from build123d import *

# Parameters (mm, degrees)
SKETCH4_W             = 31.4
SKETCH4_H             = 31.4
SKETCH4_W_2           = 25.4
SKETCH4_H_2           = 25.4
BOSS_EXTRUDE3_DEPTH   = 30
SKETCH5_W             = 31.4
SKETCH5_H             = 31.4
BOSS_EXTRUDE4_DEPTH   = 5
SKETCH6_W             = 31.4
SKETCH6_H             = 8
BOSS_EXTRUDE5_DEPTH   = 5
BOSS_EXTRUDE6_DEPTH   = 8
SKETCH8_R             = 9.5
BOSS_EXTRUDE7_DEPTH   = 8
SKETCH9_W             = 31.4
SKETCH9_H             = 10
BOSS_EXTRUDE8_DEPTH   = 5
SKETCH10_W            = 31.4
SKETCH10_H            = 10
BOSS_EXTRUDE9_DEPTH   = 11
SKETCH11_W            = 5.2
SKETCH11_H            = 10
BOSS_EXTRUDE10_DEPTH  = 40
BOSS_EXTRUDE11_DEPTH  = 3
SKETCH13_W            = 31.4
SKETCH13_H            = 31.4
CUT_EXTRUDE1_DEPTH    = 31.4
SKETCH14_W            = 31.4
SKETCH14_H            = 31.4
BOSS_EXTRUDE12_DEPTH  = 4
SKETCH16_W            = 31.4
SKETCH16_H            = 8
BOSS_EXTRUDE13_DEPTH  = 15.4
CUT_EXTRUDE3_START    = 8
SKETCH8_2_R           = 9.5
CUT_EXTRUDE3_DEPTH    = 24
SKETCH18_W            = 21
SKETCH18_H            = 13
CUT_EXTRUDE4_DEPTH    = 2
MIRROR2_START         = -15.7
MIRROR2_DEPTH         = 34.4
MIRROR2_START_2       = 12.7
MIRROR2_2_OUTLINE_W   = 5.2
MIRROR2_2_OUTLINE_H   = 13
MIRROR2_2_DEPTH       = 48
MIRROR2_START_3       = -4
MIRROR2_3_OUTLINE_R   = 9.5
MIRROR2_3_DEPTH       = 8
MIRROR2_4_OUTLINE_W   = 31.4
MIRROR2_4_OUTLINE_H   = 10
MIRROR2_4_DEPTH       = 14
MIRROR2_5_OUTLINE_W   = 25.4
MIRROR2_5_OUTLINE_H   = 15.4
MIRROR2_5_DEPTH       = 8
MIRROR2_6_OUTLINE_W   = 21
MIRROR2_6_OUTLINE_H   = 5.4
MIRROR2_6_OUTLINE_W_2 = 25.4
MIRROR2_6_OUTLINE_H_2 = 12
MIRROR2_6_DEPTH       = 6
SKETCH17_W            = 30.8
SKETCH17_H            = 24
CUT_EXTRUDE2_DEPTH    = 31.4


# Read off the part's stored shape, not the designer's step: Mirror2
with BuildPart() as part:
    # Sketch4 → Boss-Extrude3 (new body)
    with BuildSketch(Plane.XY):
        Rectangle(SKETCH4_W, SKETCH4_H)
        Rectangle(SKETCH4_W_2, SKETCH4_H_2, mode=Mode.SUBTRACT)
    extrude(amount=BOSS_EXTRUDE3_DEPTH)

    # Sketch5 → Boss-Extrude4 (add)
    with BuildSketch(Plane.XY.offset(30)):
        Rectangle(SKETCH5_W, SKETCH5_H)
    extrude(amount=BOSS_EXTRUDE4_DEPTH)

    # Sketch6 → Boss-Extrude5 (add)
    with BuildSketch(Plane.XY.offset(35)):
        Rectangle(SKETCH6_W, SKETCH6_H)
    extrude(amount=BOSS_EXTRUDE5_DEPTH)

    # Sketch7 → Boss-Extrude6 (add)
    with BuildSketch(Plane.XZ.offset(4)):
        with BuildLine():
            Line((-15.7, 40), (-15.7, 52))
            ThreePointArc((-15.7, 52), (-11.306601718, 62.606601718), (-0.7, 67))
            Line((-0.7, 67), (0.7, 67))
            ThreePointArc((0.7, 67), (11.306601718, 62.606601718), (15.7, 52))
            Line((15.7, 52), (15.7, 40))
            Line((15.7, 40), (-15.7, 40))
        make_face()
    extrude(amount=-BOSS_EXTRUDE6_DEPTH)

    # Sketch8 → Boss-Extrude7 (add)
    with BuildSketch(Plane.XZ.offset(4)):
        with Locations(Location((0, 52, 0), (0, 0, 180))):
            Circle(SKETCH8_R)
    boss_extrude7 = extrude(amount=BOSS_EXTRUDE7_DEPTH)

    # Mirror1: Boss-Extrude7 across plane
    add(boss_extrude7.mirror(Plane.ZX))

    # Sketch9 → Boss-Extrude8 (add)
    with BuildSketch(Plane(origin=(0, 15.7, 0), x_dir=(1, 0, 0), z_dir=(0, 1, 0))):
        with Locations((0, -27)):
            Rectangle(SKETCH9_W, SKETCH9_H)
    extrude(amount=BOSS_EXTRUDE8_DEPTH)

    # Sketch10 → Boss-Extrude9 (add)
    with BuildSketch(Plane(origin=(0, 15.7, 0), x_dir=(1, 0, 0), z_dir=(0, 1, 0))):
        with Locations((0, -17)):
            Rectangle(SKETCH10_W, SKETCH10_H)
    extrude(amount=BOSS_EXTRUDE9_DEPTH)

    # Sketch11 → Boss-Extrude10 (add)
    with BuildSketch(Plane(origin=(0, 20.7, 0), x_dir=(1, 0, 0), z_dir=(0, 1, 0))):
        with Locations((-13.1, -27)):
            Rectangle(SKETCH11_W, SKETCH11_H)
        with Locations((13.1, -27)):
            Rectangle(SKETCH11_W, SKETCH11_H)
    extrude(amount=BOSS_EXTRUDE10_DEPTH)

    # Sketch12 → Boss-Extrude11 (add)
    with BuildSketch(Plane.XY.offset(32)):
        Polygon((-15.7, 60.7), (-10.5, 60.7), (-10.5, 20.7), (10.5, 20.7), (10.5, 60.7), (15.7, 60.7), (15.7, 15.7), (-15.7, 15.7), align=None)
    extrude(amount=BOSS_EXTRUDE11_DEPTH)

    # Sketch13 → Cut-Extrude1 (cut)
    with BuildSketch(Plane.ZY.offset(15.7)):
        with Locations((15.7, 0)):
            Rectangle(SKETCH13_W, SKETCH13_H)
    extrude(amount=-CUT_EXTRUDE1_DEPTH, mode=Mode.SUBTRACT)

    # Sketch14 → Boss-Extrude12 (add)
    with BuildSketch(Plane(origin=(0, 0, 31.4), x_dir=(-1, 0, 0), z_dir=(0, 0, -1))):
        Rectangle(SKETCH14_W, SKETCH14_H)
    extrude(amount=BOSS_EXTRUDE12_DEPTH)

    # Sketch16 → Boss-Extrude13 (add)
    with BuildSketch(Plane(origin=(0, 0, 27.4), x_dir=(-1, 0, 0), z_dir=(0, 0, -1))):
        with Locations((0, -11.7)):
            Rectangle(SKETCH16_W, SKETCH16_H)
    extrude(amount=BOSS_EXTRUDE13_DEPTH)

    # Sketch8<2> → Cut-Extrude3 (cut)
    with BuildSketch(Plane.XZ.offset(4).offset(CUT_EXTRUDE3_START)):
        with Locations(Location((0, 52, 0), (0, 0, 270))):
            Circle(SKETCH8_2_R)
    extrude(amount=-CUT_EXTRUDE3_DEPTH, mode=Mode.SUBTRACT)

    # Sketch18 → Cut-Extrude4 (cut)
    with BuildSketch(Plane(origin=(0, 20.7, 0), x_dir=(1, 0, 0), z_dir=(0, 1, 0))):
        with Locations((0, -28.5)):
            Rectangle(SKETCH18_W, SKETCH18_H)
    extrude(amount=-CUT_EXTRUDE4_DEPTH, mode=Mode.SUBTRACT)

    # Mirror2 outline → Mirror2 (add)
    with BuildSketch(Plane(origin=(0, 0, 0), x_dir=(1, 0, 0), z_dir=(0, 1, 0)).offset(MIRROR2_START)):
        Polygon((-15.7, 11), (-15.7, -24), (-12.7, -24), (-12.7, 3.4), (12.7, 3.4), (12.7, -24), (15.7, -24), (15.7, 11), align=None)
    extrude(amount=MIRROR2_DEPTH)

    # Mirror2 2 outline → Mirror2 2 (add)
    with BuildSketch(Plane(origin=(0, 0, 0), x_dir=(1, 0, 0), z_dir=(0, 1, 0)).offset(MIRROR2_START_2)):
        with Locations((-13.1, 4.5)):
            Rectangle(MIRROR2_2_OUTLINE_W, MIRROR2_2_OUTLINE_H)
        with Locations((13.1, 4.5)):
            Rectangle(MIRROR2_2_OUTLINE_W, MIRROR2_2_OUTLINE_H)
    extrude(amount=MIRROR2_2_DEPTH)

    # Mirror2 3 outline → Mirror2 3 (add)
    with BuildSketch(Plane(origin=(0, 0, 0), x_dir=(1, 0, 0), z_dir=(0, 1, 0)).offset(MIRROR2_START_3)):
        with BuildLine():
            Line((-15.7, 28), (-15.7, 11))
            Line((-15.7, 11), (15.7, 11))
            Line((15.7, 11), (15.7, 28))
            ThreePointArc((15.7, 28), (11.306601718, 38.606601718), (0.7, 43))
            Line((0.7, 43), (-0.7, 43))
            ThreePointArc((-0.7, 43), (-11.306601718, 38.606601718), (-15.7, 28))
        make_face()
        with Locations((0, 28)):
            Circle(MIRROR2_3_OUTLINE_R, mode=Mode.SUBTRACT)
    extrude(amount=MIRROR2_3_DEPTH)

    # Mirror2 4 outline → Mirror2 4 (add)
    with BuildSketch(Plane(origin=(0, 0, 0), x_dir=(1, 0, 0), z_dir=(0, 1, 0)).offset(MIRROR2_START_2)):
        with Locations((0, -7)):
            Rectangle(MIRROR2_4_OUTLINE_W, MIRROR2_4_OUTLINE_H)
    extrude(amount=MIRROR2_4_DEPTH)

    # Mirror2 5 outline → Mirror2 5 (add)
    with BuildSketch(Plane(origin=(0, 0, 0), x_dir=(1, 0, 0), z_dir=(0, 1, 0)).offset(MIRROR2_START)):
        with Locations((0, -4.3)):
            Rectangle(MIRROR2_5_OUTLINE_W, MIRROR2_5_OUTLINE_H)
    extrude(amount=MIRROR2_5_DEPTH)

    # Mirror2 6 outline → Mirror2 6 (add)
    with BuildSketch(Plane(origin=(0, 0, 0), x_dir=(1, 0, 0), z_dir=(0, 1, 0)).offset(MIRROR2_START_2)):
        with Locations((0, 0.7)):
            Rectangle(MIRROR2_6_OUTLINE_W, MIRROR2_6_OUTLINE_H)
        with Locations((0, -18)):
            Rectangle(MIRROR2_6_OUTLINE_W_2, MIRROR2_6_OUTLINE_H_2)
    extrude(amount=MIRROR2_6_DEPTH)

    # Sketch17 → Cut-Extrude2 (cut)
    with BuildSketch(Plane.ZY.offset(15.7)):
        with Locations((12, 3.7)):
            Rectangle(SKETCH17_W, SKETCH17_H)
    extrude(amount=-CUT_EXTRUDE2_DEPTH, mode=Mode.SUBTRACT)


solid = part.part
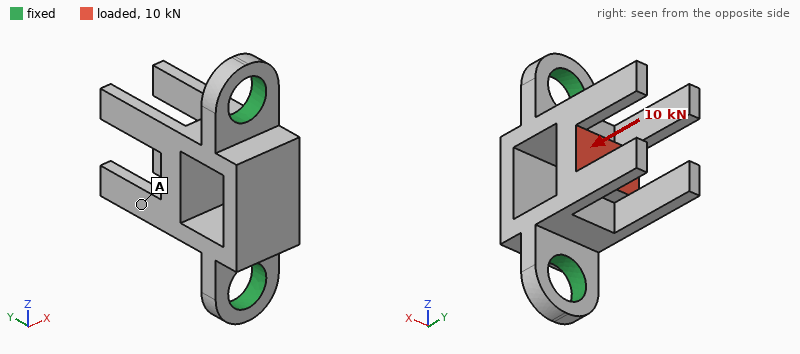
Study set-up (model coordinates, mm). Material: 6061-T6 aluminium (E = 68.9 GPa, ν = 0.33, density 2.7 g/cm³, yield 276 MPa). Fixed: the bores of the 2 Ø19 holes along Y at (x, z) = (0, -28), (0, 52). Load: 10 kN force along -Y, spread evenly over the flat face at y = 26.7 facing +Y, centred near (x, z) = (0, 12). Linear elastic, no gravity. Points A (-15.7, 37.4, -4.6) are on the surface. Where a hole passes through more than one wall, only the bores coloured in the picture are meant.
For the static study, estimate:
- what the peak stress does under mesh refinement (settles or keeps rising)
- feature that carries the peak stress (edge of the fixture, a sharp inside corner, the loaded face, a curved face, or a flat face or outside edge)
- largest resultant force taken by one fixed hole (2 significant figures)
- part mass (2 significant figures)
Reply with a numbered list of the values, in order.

1. keeps rising
2. edge of the fixture
3. 5.3 kN
4. 140 g
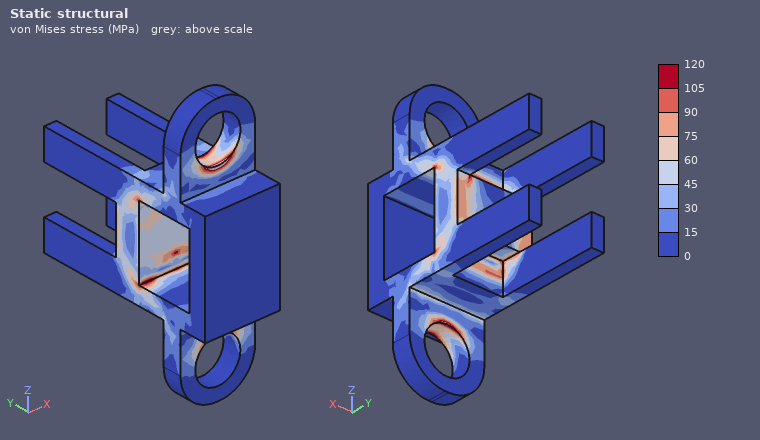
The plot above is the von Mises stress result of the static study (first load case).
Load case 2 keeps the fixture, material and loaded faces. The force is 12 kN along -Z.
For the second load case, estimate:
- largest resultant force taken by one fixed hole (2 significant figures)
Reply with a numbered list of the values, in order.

1. 8.0 kN
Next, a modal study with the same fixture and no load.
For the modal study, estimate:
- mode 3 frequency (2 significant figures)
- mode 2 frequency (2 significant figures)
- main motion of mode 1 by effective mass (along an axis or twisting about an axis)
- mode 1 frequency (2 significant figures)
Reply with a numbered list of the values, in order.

1. 2500 Hz
2. 2500 Hz
3. along X
4. 2100 Hz
